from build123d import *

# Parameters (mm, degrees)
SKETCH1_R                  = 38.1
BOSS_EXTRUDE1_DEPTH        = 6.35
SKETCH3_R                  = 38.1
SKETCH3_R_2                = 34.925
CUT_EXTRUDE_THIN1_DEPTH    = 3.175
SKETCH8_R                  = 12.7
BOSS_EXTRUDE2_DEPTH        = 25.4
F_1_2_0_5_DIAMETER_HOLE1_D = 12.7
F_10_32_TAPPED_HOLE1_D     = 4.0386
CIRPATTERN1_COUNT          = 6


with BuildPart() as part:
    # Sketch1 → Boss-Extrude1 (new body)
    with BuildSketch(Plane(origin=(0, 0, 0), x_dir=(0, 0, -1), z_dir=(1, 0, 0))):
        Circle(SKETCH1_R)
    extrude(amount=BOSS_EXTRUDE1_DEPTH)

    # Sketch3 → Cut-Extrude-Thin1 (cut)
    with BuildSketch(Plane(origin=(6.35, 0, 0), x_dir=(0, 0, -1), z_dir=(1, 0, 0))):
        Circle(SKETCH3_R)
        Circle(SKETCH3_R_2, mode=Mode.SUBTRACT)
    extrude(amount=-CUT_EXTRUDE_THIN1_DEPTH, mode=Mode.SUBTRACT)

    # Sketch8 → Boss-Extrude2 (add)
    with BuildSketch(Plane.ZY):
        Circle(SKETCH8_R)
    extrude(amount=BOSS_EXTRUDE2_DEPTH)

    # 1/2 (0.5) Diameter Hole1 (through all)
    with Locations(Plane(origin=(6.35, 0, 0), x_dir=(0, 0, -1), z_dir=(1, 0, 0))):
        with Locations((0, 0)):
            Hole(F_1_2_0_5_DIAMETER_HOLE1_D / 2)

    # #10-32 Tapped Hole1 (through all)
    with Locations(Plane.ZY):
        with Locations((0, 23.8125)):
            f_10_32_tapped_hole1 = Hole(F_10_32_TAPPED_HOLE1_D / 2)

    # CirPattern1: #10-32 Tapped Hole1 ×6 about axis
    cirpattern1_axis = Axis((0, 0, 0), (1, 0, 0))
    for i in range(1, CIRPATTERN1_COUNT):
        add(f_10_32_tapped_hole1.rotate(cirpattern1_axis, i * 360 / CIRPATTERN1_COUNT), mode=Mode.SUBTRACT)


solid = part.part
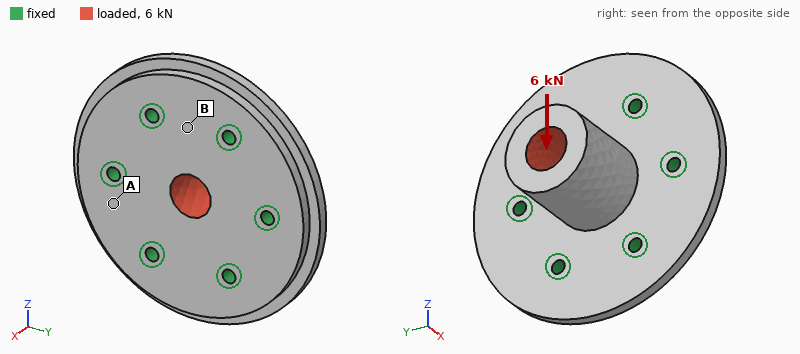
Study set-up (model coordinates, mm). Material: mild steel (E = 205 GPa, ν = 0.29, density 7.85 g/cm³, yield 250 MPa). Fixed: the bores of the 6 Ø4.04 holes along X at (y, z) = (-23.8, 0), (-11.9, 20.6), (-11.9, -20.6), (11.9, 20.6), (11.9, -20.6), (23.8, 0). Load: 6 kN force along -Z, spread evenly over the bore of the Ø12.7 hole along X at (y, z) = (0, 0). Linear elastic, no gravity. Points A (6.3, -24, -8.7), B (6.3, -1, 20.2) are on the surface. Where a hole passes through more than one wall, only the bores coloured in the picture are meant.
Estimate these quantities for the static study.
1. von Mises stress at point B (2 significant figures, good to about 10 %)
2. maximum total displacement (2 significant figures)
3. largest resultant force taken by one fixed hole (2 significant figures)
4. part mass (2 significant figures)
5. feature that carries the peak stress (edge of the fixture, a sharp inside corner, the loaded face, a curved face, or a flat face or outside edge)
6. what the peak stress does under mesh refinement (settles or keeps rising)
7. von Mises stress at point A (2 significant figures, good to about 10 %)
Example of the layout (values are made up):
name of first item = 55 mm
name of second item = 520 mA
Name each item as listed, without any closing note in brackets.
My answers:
von Mises stress at point B = 21 MPa
maximum total displacement = 18 µm
largest resultant force taken by one fixed hole = 1.7 kN
part mass = 270 g
feature that carries the peak stress = edge of the fixture
what the peak stress does under mesh refinement = keeps rising
von Mises stress at point A = 9.6 MPa
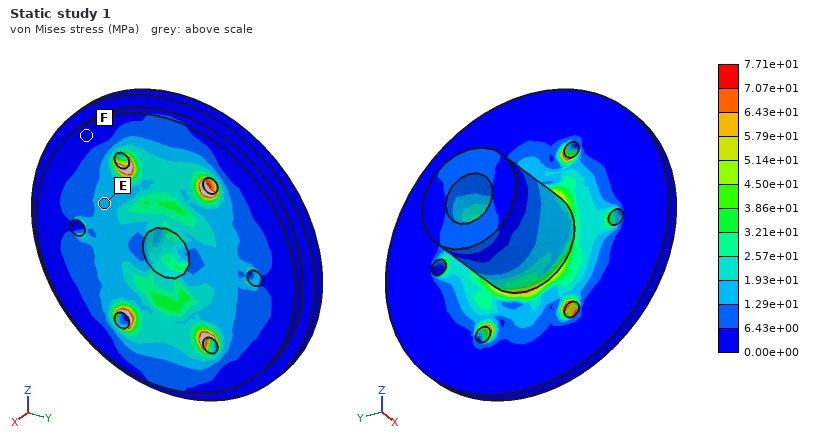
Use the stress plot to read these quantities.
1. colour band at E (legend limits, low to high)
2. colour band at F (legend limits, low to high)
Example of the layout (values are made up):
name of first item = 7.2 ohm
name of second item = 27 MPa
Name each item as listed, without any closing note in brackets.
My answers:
colour band at E = 1.29e+01 to 1.93e+01 MPa
colour band at F = 0.00e+00 to 6.43e+00 MPa
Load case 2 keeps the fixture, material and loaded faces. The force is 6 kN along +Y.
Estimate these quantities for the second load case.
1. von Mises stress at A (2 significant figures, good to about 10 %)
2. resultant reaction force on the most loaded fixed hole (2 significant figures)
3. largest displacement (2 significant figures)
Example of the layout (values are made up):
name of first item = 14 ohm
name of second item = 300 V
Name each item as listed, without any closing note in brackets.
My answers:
von Mises stress at A = 16 MPa
resultant reaction force on the most loaded fixed hole = 2.0 kN
largest displacement = 18 µm
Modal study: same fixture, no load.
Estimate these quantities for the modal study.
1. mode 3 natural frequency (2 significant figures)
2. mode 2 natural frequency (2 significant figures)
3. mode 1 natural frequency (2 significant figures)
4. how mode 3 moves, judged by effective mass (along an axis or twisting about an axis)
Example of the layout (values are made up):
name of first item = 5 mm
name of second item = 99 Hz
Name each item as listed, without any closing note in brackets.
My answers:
mode 3 natural frequency = 15 kHz
mode 2 natural frequency = 11 kHz
mode 1 natural frequency = 11 kHz
how mode 3 moves, judged by effective mass = along X
